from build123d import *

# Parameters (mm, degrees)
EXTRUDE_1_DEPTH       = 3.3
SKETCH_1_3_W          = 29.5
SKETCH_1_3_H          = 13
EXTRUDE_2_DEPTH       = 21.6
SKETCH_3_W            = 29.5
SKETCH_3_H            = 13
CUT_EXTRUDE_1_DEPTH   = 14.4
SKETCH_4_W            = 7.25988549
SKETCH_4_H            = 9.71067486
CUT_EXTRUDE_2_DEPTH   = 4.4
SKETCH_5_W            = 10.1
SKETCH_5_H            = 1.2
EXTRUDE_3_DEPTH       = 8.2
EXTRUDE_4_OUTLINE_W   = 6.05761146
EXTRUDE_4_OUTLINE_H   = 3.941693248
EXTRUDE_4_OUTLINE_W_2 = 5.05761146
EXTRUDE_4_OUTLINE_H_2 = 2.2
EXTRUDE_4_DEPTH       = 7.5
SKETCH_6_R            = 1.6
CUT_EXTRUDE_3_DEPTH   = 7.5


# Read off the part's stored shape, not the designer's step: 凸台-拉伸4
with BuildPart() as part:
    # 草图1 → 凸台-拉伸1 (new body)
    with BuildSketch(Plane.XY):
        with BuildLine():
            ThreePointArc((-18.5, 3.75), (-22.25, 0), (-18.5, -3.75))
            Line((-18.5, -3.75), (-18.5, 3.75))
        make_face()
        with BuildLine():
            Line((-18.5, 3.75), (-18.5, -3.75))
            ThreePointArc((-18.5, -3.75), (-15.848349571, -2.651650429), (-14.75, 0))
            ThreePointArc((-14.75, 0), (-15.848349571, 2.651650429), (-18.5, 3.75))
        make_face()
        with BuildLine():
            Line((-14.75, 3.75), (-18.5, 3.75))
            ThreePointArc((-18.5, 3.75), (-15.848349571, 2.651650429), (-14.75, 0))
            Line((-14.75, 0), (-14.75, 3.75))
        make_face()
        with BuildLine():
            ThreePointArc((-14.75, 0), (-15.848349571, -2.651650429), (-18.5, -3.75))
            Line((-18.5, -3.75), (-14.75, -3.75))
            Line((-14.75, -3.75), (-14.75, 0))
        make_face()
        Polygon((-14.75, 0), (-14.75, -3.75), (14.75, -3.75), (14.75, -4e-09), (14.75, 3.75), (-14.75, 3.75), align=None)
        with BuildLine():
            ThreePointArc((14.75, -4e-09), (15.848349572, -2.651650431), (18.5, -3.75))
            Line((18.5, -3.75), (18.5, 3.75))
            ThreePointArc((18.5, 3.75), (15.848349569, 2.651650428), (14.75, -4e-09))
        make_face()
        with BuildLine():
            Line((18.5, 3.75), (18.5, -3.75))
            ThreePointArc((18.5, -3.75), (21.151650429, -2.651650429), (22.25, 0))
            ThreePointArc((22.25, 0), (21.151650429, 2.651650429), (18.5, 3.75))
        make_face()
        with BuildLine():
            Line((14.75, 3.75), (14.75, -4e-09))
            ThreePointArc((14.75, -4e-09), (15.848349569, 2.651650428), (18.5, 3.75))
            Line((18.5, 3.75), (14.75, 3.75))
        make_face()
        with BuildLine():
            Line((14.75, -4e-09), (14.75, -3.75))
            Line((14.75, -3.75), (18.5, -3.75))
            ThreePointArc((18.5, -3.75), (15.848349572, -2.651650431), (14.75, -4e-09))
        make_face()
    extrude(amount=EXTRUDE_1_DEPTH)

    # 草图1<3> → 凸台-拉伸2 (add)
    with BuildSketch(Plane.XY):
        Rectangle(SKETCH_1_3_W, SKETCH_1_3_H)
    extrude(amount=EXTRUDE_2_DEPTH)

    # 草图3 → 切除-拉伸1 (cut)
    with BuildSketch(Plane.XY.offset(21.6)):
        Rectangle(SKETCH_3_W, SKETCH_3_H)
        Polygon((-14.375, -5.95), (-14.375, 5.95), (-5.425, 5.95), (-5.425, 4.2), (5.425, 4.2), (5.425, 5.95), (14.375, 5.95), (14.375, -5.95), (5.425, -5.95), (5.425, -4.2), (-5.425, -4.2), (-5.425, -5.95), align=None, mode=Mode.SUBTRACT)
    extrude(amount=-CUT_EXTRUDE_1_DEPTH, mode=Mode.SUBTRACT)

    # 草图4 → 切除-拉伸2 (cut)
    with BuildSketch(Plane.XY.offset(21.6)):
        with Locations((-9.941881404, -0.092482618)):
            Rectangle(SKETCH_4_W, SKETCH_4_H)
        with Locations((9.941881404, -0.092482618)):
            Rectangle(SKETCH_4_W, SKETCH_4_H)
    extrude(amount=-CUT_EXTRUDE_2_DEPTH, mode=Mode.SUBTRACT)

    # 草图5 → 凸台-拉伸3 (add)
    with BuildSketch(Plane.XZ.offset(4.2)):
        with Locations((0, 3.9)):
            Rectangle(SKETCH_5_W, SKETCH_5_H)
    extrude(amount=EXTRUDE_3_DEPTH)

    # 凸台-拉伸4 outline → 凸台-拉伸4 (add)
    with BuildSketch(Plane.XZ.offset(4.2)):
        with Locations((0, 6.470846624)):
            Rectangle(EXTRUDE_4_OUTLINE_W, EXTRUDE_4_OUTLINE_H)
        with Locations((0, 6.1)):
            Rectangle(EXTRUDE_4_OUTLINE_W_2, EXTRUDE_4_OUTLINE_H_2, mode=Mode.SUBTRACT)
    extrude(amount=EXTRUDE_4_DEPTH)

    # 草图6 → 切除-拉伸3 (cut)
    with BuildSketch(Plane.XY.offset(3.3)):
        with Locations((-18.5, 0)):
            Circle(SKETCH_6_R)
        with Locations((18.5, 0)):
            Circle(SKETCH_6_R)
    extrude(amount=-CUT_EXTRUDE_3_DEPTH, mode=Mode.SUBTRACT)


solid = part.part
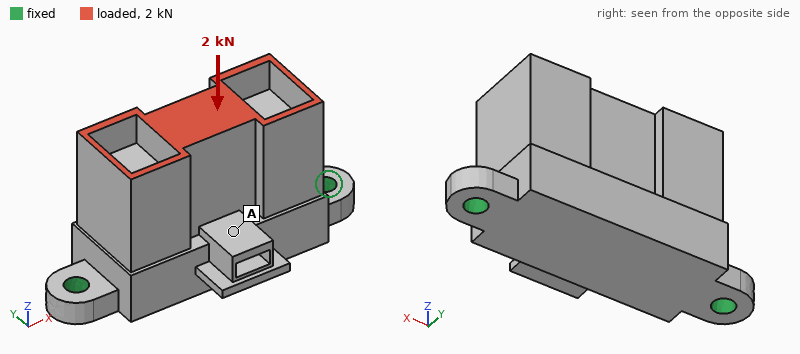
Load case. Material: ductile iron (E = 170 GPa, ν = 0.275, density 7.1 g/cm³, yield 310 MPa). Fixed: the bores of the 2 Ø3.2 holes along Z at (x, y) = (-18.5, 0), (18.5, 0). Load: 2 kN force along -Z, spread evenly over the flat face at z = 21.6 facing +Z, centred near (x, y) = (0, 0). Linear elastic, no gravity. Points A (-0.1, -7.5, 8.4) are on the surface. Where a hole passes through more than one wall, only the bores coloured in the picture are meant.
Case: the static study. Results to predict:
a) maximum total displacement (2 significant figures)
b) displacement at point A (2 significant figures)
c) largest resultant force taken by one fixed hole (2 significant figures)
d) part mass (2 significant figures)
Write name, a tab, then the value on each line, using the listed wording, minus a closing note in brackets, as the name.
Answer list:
maximum total displacement	7.0 µm
displacement at point A	5.7 µm
largest resultant force taken by one fixed hole	1.1 kN
part mass	49 g
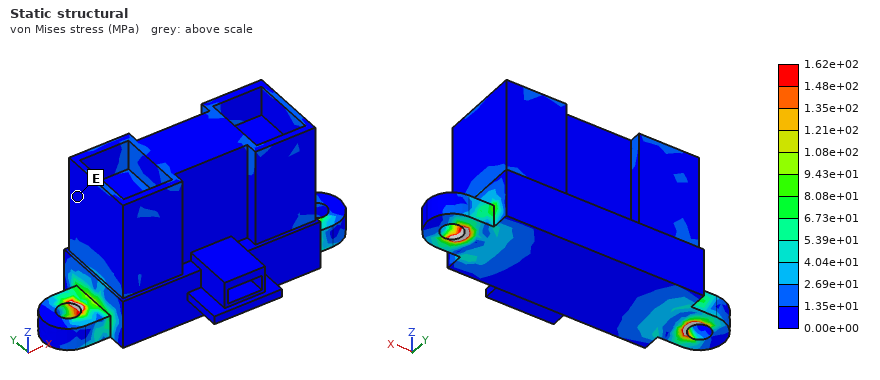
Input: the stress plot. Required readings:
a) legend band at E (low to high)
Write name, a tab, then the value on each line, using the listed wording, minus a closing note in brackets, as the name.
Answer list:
legend band at E	0.00e+00 to 1.35e+01 MPa
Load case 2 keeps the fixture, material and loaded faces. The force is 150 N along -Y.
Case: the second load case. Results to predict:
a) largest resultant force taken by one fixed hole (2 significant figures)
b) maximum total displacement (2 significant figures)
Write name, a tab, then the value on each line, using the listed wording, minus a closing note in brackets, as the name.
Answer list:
largest resultant force taken by one fixed hole	75 N
maximum total displacement	24 µm
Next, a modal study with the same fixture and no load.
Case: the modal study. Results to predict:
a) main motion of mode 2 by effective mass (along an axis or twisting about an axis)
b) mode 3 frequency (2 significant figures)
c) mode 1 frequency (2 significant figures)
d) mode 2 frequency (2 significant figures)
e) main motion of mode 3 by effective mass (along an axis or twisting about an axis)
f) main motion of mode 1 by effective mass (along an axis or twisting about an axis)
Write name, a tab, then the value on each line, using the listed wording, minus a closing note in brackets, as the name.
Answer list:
main motion of mode 2 by effective mass	along Z
mode 3 frequency	17 kHz
mode 1 frequency	3700 Hz
mode 2 frequency	14 kHz
main motion of mode 3 by effective mass	along X
main motion of mode 1 by effective mass	along Y
